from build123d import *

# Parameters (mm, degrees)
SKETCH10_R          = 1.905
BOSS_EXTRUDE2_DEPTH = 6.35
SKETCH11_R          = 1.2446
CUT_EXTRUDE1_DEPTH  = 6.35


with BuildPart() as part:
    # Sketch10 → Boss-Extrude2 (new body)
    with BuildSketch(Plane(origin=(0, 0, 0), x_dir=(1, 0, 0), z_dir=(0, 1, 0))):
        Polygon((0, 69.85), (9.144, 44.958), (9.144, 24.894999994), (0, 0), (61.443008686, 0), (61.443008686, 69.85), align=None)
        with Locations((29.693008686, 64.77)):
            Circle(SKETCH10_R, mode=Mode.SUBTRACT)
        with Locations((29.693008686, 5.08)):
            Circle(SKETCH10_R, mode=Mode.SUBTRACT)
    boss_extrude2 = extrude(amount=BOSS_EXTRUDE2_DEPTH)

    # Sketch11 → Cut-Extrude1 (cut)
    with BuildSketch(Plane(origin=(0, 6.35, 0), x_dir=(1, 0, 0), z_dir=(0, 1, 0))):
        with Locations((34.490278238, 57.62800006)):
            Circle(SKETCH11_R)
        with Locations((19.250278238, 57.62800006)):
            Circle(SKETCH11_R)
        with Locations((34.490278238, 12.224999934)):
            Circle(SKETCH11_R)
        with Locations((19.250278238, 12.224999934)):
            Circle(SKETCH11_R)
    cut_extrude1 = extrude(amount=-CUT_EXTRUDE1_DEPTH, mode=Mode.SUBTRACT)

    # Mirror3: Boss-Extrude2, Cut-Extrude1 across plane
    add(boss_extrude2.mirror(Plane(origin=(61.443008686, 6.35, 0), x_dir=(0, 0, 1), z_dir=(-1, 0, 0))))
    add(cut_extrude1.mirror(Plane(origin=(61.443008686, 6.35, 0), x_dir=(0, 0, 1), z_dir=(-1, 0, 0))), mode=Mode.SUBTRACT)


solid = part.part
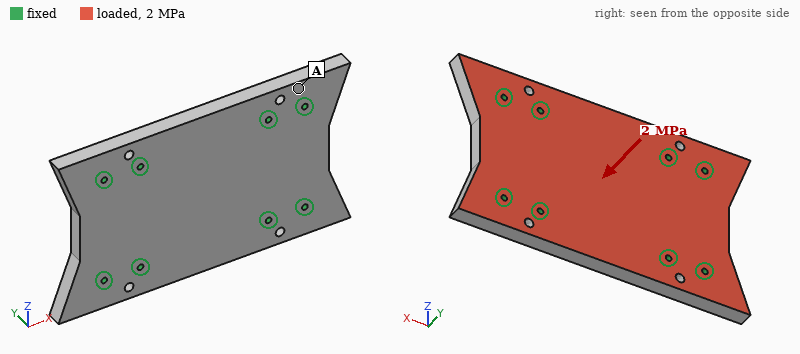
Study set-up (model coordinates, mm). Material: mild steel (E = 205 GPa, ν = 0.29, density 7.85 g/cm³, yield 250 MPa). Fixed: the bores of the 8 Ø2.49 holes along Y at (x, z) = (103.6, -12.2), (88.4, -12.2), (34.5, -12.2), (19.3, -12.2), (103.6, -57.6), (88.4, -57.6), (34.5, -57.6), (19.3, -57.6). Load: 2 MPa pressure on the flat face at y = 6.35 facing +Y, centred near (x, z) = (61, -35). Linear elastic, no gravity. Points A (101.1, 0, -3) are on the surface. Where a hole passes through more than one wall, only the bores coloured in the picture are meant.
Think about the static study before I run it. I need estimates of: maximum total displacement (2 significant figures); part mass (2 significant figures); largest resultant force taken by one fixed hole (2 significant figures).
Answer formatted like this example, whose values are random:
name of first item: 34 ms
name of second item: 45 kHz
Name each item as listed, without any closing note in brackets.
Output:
maximum total displacement: 23 µm
part mass: 380 g
largest resultant force taken by one fixed hole: 2.6 kN
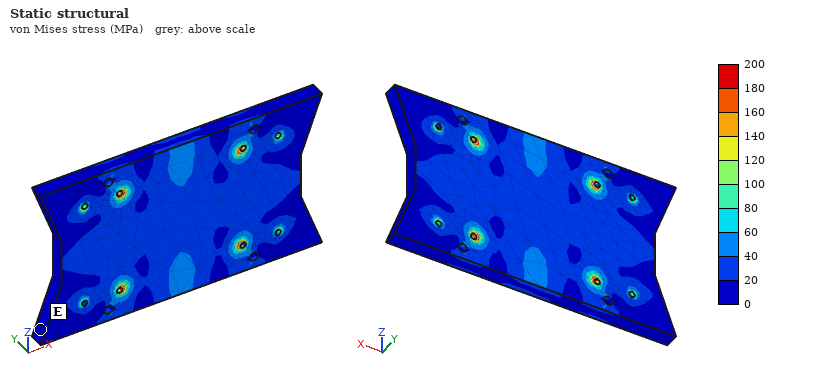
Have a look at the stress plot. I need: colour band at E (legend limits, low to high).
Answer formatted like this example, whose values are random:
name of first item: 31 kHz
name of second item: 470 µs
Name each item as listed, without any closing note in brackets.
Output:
colour band at E: 0 to 20 MPa
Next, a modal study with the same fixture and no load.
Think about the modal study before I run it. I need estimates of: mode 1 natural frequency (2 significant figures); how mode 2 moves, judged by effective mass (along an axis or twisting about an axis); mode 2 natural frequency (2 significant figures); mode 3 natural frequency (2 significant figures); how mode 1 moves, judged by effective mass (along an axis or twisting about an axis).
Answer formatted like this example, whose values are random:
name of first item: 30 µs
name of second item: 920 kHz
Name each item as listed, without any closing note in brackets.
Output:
mode 1 natural frequency: 7900 Hz
how mode 2 moves, judged by effective mass: twisting about X
mode 2 natural frequency: 10000 Hz
mode 3 natural frequency: 11 kHz
how mode 1 moves, judged by effective mass: along Y
